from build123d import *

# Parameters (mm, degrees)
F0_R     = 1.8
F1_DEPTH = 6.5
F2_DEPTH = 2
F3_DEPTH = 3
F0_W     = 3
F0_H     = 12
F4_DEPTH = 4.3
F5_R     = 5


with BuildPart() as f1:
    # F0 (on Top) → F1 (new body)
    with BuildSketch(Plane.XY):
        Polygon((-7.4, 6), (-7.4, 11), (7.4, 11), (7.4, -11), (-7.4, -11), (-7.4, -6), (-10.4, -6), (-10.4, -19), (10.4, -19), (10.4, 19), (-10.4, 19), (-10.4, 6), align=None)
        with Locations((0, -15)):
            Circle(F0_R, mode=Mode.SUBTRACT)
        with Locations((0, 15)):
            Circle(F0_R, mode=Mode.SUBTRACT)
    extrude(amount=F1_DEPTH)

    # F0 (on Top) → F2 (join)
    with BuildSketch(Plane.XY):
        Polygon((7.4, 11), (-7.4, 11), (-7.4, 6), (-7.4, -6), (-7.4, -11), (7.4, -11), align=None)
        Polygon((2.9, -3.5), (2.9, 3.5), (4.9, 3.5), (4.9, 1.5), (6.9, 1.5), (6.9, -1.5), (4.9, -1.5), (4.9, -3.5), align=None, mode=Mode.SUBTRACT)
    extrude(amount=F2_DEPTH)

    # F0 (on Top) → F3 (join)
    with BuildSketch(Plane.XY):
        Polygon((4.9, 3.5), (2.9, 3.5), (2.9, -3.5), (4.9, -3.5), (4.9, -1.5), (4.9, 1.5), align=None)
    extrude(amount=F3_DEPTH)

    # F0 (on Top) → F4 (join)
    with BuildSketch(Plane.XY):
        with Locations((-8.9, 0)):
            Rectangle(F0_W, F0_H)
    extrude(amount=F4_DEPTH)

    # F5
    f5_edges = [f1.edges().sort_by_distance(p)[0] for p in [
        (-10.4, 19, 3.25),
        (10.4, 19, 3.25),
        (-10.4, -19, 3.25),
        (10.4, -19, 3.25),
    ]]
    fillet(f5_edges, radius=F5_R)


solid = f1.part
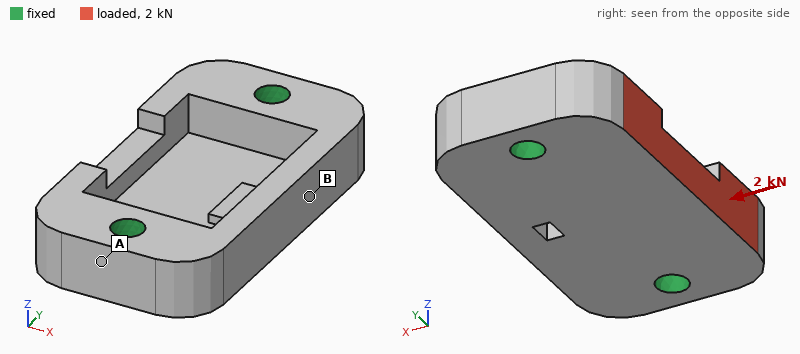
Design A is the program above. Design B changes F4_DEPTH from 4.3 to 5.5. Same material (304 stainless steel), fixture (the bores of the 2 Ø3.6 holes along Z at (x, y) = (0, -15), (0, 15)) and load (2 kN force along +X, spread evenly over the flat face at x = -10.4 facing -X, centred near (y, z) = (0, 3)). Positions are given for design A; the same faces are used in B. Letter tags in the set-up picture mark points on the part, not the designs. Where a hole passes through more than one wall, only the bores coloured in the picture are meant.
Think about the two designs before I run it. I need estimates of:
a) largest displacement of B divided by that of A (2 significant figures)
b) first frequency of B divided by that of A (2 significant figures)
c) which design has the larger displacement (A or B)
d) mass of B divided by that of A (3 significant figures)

1.5
1.0
B
1.01
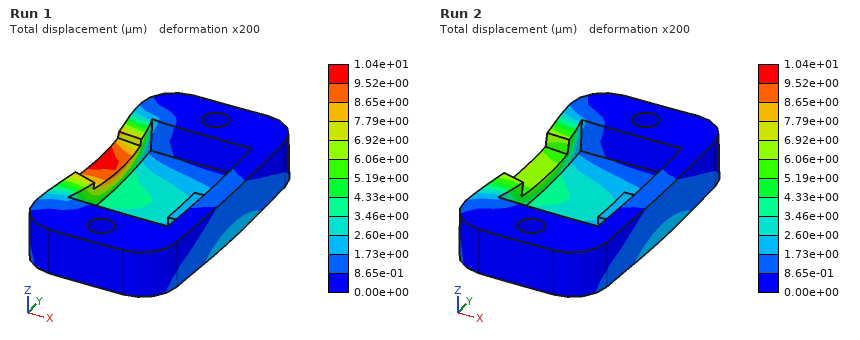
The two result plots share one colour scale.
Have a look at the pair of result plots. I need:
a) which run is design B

Run 1
